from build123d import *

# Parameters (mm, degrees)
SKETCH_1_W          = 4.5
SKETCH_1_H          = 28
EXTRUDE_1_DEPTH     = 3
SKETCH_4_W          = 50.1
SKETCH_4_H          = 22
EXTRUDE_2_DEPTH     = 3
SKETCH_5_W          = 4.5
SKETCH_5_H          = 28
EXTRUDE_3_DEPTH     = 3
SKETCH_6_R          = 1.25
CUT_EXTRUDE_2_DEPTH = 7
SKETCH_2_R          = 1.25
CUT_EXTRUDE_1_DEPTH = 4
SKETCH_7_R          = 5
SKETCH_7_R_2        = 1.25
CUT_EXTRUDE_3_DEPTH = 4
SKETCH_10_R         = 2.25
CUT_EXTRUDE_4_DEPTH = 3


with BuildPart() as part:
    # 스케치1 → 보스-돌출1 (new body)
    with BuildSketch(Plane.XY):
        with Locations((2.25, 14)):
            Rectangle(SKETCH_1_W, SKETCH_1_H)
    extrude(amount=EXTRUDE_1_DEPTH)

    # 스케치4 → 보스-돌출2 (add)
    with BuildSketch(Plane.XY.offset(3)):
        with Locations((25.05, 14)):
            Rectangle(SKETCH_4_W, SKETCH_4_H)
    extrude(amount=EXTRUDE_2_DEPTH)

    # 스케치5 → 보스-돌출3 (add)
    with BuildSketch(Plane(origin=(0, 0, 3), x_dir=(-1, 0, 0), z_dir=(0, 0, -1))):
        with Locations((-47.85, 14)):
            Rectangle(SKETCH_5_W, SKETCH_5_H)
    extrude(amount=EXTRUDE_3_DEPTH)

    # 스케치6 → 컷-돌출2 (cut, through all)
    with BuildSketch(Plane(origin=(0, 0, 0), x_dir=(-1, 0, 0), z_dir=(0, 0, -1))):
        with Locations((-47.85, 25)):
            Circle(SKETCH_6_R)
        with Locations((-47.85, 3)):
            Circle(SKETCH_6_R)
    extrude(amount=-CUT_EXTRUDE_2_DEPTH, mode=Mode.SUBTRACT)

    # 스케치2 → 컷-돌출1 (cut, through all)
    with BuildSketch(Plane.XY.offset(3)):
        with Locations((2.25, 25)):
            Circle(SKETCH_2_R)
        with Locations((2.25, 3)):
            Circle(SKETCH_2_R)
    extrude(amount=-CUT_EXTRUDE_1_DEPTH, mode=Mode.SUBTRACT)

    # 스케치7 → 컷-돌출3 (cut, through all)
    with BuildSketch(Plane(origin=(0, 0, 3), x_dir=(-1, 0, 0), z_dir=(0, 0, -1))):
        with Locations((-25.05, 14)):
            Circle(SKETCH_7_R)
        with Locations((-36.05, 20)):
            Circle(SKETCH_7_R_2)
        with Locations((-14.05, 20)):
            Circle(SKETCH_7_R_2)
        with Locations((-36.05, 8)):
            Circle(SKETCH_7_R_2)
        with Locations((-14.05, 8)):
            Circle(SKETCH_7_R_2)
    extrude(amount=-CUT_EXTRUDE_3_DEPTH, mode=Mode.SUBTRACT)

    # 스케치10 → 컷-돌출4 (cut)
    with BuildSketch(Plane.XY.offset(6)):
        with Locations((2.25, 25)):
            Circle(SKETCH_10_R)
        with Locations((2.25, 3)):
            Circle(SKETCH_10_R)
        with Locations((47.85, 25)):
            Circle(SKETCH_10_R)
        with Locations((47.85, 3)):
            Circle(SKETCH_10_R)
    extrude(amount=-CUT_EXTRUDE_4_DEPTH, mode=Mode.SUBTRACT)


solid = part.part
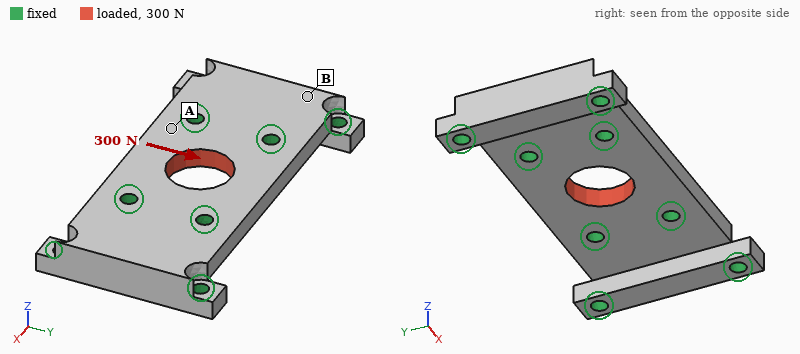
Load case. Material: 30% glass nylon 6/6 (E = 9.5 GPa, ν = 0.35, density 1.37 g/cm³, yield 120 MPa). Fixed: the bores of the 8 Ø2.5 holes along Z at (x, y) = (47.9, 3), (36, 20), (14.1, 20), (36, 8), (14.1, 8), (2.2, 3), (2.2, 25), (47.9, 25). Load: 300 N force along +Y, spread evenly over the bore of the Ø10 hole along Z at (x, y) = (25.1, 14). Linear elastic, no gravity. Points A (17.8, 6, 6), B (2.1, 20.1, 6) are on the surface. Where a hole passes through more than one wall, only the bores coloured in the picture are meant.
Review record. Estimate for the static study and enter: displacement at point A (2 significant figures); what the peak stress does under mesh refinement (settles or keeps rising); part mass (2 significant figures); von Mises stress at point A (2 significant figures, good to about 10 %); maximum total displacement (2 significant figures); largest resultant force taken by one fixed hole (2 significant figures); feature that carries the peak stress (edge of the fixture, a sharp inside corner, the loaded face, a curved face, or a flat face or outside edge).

3.0 µm
keeps rising
5.0 g
3.3 MPa
8.6 µm
83 N
edge of the fixture
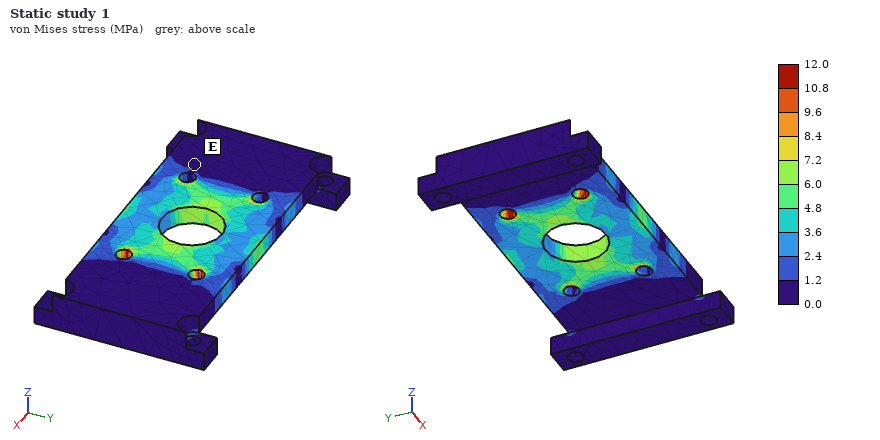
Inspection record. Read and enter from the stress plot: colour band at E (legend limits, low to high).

0.0 to 1.2 MPa
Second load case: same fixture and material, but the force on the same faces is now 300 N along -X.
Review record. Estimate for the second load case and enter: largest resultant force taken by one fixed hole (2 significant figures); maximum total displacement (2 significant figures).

75 N
3.3 µm
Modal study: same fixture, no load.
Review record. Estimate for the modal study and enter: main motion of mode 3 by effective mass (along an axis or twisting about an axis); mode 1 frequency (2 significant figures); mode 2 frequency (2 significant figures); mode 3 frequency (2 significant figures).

twisting about Y
16 kHz
17 kHz
21 kHz
